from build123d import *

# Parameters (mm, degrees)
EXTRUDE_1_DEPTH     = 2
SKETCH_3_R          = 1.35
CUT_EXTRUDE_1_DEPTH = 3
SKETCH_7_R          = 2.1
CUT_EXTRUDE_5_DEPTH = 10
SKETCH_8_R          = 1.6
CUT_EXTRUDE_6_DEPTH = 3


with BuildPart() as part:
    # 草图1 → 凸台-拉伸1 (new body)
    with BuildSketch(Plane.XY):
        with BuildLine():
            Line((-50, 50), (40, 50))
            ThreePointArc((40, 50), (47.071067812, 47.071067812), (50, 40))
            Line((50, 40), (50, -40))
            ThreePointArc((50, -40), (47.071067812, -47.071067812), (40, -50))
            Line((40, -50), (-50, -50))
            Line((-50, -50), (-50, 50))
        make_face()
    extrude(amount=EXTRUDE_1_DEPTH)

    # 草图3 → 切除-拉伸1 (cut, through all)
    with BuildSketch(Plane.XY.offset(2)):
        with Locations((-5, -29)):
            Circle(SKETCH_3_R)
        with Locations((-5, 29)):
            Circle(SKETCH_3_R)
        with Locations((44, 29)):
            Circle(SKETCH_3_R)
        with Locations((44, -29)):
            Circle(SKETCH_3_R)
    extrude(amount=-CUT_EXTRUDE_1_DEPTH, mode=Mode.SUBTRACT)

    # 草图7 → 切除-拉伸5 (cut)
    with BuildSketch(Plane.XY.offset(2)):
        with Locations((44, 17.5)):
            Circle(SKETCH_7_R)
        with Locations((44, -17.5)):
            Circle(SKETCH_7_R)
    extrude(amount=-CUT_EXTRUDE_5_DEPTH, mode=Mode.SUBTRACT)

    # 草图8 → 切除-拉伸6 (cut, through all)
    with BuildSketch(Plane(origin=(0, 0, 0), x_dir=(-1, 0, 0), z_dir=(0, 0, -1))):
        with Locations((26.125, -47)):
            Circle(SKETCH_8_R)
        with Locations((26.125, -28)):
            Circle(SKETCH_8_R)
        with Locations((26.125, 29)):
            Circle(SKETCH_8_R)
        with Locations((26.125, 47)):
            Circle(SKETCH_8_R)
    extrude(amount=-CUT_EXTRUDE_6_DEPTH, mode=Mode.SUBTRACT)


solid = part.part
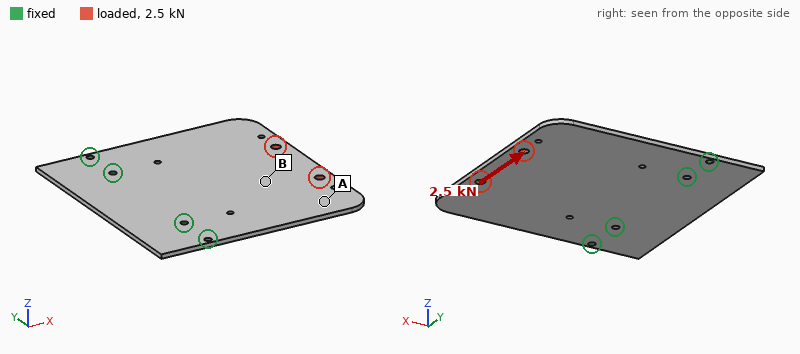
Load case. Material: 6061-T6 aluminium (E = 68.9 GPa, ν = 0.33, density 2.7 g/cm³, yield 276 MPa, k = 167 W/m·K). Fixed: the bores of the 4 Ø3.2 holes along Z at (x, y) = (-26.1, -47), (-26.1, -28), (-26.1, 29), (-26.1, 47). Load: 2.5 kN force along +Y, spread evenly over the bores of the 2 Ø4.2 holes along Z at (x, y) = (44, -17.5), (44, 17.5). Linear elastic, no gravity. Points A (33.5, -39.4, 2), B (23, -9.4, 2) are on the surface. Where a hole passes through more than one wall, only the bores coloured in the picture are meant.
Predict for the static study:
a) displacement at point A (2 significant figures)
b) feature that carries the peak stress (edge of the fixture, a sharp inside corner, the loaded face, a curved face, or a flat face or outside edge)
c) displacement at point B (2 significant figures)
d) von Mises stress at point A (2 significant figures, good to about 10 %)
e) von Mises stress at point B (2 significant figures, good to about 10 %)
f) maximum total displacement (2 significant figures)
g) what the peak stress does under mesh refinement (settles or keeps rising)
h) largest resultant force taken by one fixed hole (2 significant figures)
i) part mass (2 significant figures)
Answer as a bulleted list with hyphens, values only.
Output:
- 60 µm
- edge of the fixture
- 44 µm
- 13 MPa
- 31 MPa
- 75 µm
- keeps rising
- 1.4 kN
- 53 g
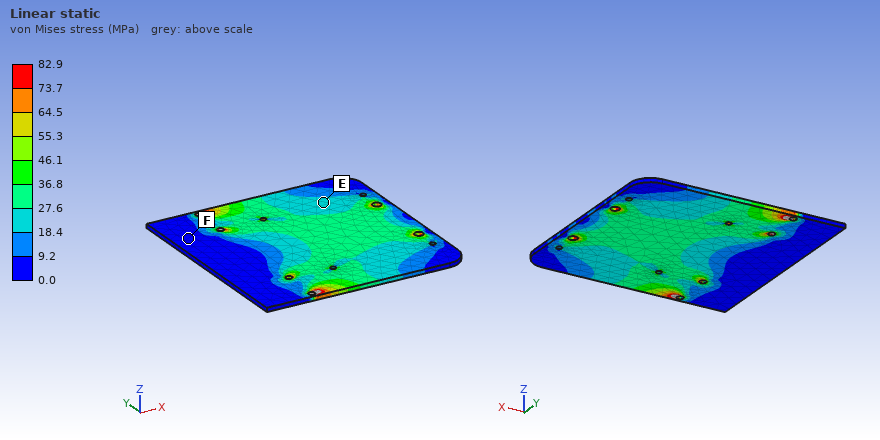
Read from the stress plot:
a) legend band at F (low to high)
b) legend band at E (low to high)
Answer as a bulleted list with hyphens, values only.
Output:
- 0.0 to 9.2 MPa
- 18.4 to 27.6 MPa
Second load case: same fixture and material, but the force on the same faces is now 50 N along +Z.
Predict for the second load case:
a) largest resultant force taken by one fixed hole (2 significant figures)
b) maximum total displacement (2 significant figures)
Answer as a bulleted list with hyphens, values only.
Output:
- 34 N
- 1.6 mm
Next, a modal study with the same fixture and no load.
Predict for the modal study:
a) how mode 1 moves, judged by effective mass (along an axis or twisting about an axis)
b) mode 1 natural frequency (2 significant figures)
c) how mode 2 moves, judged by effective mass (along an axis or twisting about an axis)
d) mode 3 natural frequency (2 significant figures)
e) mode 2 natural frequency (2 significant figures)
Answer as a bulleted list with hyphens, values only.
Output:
- along Z
- 270 Hz
- twisting about X
- 1400 Hz
- 590 Hz
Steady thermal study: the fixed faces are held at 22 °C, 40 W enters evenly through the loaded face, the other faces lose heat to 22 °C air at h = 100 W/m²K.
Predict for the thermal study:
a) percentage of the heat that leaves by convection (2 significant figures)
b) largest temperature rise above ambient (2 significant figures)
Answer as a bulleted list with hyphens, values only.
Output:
- 76 %
- 61 K
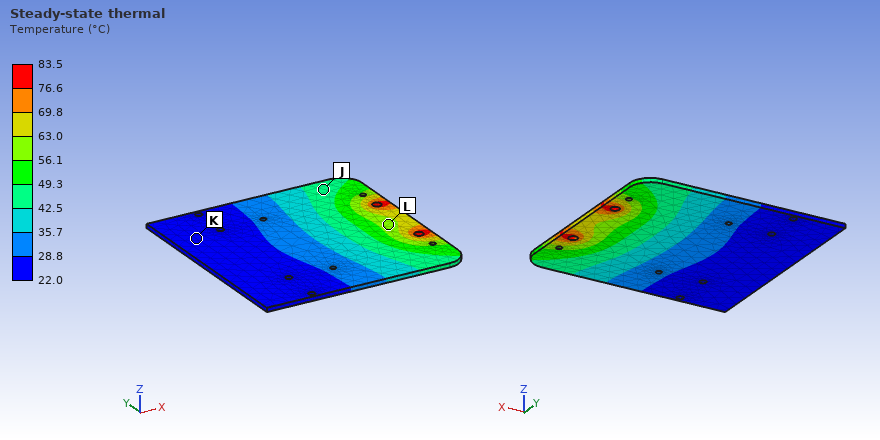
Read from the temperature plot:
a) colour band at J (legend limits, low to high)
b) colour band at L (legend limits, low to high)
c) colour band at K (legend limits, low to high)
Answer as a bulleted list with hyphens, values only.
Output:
- 42.5 to 49.3 °C
- 56.1 to 63.0 °C
- 22.0 to 28.8 °C
